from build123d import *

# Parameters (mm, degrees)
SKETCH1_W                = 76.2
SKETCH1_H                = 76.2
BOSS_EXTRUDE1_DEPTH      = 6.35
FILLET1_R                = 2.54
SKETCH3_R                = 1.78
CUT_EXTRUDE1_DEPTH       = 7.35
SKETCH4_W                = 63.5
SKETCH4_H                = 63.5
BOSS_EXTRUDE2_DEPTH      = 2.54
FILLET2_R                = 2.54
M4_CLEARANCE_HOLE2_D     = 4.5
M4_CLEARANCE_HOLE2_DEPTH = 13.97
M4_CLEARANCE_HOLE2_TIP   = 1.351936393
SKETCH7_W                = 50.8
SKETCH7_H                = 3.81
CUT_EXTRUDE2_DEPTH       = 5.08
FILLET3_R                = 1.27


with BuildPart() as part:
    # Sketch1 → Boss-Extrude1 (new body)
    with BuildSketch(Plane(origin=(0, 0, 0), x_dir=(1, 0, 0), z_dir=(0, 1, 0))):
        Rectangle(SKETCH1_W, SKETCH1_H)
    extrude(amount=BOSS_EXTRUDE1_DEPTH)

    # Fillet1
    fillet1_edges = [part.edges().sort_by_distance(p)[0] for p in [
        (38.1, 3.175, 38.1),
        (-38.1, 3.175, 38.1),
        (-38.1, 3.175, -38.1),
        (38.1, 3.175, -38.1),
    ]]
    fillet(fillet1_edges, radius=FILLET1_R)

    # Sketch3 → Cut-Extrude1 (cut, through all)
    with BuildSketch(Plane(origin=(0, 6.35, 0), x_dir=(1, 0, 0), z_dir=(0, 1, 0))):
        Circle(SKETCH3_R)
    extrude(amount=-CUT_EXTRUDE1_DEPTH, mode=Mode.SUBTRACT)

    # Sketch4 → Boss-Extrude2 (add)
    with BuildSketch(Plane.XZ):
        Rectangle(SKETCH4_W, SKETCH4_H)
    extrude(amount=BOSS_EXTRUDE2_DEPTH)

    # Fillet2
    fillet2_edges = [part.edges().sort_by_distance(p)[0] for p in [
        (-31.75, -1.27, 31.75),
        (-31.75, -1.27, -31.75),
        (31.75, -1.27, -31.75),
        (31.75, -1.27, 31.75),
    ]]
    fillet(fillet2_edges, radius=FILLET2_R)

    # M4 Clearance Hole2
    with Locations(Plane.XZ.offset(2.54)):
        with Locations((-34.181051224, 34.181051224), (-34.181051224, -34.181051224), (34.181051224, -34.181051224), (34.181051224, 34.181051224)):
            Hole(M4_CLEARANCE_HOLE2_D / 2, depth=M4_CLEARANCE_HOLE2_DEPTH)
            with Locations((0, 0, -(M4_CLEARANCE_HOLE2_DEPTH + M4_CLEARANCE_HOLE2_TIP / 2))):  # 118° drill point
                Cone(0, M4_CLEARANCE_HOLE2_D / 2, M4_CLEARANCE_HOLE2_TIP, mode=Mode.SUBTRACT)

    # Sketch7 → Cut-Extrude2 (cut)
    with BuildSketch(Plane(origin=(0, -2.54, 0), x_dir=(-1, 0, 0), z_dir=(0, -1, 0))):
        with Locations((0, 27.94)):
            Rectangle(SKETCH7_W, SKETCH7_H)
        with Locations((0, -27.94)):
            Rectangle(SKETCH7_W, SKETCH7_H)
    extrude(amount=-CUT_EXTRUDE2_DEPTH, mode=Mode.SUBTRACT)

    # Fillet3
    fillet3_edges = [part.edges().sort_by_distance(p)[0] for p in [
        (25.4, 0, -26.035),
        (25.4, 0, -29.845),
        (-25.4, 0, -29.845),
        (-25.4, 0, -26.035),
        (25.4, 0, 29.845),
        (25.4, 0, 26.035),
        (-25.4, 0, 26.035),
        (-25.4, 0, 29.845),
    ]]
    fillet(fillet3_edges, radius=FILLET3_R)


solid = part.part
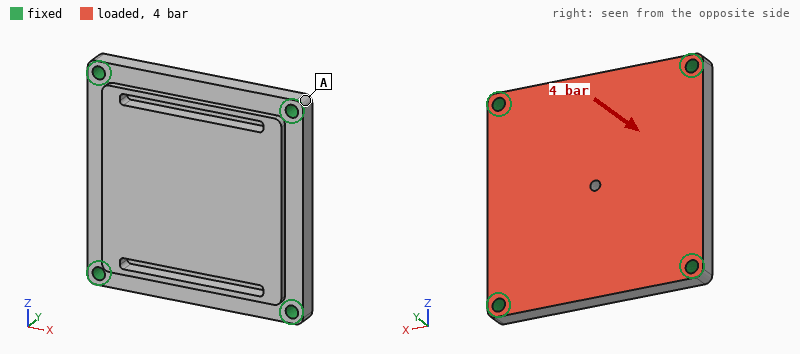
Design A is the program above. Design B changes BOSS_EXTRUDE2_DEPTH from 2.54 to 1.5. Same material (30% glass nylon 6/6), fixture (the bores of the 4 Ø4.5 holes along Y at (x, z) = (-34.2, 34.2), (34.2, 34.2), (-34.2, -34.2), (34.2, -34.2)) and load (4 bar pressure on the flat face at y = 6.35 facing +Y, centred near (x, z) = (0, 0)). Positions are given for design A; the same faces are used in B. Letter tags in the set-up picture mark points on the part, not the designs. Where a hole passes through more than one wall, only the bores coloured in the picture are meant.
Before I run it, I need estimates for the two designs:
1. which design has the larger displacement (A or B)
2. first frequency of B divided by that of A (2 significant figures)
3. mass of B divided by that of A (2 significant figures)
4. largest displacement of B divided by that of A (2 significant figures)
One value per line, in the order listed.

B
0.96
0.92
1.2
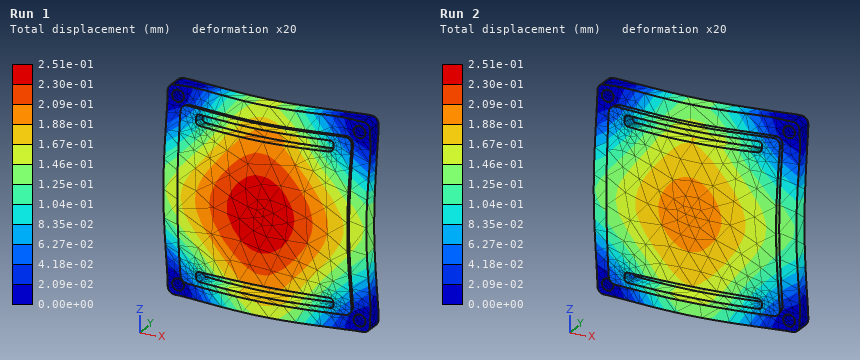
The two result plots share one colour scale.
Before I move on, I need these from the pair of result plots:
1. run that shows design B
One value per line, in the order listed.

Run 1
